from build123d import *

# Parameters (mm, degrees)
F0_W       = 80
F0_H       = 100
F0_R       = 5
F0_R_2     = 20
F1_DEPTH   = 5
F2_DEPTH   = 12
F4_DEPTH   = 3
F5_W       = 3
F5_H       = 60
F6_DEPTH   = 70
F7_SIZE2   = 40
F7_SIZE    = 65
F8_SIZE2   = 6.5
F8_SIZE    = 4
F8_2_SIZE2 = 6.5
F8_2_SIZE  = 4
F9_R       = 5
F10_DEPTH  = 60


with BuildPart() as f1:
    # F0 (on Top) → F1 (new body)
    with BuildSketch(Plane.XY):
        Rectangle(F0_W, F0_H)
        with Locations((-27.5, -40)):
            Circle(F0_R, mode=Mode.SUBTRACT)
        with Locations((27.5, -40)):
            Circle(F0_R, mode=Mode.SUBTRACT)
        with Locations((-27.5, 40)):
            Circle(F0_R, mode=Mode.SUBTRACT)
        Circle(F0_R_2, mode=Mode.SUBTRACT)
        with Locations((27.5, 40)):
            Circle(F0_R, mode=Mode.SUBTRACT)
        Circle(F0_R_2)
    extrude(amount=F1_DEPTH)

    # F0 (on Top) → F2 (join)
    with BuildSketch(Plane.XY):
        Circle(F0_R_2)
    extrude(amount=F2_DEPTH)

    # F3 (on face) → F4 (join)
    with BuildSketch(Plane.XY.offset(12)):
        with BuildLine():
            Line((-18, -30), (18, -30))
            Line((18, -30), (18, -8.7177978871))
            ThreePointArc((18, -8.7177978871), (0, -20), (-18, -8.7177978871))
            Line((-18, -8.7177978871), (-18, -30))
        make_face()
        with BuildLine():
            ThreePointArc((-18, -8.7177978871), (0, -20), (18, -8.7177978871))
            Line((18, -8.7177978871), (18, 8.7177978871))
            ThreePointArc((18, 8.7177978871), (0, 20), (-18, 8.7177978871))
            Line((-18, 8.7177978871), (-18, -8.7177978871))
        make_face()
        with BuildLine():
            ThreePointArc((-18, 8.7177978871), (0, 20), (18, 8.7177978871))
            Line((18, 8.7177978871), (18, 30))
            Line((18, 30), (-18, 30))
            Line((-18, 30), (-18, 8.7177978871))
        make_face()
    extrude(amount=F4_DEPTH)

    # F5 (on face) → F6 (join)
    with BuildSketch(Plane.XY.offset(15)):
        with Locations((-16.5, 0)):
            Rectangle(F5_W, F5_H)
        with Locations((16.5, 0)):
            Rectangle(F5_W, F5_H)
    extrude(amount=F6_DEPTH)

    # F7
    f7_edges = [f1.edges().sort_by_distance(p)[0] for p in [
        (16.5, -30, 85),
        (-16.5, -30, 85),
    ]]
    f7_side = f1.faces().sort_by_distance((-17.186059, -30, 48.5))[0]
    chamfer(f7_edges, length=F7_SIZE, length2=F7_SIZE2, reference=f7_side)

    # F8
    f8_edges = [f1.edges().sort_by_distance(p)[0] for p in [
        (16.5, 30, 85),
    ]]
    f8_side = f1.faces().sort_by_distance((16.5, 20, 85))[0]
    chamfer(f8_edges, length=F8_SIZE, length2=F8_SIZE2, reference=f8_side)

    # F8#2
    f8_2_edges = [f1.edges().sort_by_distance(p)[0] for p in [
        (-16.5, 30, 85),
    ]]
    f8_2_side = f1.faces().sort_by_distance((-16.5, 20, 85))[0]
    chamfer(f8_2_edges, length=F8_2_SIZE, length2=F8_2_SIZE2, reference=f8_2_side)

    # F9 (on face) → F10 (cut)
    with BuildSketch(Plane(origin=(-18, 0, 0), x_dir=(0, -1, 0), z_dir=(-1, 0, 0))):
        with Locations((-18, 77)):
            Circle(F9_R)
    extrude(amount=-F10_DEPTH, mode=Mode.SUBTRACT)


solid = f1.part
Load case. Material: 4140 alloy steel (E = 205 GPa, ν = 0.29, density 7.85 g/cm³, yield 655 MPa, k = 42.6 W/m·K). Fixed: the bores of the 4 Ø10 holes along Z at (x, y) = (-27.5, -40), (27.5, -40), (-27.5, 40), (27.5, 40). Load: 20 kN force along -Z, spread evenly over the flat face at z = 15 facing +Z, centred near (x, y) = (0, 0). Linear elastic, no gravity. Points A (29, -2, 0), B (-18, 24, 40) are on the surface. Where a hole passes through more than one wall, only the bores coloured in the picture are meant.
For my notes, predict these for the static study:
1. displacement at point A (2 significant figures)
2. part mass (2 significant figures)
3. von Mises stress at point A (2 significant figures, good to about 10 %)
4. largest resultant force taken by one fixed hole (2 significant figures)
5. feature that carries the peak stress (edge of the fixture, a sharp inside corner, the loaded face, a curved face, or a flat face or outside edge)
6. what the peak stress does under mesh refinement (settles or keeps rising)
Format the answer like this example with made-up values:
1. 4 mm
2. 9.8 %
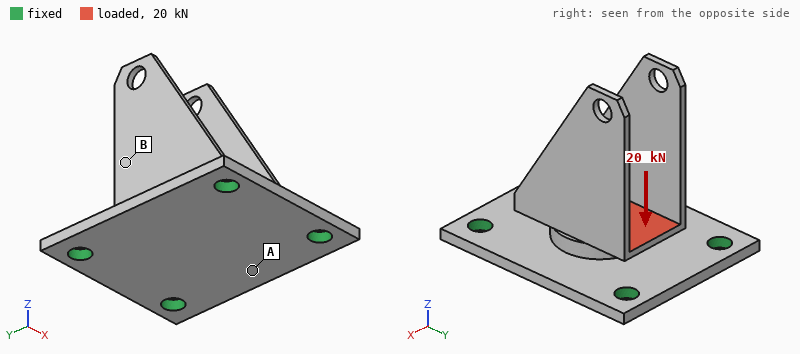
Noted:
1. 0.13 mm
2. 550 g
3. 160 MPa
4. 5.3 kN
5. edge of the fixture
6. keeps rising
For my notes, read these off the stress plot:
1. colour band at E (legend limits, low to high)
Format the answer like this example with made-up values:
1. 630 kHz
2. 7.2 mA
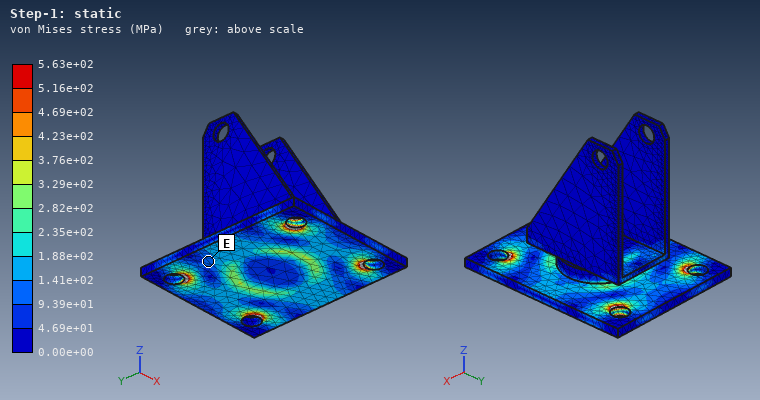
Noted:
1. 9.39e+01 to 1.41e+02 MPa
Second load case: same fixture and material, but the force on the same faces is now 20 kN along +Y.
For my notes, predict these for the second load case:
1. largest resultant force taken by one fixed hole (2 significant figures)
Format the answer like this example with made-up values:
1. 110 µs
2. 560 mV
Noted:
1. 5.7 kN
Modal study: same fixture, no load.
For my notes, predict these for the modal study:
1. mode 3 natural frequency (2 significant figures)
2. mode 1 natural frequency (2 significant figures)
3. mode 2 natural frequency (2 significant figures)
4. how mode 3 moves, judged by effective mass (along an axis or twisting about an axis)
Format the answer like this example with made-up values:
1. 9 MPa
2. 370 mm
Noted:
1. 2300 Hz
2. 650 Hz
3. 670 Hz
4. along Y
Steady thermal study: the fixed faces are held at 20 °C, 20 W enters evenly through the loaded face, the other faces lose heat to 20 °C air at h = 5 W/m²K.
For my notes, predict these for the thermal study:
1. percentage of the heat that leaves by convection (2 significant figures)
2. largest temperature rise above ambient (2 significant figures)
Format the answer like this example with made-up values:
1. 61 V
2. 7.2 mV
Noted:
1. 11 %
2. 29 K
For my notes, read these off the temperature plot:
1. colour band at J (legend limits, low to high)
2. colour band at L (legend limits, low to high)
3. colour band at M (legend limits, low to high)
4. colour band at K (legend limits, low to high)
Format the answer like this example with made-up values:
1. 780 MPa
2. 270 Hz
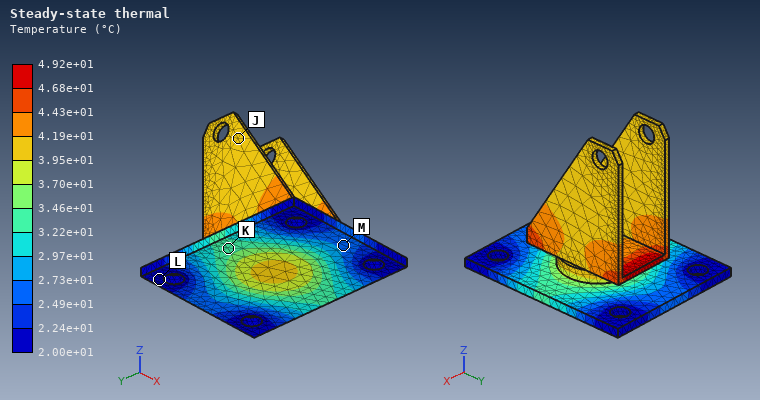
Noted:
1. 3.95e+01 to 4.19e+01 °C
2. 2.00e+01 to 2.24e+01 °C
3. 2.49e+01 to 2.73e+01 °C
4. 3.22e+01 to 3.46e+01 °C
